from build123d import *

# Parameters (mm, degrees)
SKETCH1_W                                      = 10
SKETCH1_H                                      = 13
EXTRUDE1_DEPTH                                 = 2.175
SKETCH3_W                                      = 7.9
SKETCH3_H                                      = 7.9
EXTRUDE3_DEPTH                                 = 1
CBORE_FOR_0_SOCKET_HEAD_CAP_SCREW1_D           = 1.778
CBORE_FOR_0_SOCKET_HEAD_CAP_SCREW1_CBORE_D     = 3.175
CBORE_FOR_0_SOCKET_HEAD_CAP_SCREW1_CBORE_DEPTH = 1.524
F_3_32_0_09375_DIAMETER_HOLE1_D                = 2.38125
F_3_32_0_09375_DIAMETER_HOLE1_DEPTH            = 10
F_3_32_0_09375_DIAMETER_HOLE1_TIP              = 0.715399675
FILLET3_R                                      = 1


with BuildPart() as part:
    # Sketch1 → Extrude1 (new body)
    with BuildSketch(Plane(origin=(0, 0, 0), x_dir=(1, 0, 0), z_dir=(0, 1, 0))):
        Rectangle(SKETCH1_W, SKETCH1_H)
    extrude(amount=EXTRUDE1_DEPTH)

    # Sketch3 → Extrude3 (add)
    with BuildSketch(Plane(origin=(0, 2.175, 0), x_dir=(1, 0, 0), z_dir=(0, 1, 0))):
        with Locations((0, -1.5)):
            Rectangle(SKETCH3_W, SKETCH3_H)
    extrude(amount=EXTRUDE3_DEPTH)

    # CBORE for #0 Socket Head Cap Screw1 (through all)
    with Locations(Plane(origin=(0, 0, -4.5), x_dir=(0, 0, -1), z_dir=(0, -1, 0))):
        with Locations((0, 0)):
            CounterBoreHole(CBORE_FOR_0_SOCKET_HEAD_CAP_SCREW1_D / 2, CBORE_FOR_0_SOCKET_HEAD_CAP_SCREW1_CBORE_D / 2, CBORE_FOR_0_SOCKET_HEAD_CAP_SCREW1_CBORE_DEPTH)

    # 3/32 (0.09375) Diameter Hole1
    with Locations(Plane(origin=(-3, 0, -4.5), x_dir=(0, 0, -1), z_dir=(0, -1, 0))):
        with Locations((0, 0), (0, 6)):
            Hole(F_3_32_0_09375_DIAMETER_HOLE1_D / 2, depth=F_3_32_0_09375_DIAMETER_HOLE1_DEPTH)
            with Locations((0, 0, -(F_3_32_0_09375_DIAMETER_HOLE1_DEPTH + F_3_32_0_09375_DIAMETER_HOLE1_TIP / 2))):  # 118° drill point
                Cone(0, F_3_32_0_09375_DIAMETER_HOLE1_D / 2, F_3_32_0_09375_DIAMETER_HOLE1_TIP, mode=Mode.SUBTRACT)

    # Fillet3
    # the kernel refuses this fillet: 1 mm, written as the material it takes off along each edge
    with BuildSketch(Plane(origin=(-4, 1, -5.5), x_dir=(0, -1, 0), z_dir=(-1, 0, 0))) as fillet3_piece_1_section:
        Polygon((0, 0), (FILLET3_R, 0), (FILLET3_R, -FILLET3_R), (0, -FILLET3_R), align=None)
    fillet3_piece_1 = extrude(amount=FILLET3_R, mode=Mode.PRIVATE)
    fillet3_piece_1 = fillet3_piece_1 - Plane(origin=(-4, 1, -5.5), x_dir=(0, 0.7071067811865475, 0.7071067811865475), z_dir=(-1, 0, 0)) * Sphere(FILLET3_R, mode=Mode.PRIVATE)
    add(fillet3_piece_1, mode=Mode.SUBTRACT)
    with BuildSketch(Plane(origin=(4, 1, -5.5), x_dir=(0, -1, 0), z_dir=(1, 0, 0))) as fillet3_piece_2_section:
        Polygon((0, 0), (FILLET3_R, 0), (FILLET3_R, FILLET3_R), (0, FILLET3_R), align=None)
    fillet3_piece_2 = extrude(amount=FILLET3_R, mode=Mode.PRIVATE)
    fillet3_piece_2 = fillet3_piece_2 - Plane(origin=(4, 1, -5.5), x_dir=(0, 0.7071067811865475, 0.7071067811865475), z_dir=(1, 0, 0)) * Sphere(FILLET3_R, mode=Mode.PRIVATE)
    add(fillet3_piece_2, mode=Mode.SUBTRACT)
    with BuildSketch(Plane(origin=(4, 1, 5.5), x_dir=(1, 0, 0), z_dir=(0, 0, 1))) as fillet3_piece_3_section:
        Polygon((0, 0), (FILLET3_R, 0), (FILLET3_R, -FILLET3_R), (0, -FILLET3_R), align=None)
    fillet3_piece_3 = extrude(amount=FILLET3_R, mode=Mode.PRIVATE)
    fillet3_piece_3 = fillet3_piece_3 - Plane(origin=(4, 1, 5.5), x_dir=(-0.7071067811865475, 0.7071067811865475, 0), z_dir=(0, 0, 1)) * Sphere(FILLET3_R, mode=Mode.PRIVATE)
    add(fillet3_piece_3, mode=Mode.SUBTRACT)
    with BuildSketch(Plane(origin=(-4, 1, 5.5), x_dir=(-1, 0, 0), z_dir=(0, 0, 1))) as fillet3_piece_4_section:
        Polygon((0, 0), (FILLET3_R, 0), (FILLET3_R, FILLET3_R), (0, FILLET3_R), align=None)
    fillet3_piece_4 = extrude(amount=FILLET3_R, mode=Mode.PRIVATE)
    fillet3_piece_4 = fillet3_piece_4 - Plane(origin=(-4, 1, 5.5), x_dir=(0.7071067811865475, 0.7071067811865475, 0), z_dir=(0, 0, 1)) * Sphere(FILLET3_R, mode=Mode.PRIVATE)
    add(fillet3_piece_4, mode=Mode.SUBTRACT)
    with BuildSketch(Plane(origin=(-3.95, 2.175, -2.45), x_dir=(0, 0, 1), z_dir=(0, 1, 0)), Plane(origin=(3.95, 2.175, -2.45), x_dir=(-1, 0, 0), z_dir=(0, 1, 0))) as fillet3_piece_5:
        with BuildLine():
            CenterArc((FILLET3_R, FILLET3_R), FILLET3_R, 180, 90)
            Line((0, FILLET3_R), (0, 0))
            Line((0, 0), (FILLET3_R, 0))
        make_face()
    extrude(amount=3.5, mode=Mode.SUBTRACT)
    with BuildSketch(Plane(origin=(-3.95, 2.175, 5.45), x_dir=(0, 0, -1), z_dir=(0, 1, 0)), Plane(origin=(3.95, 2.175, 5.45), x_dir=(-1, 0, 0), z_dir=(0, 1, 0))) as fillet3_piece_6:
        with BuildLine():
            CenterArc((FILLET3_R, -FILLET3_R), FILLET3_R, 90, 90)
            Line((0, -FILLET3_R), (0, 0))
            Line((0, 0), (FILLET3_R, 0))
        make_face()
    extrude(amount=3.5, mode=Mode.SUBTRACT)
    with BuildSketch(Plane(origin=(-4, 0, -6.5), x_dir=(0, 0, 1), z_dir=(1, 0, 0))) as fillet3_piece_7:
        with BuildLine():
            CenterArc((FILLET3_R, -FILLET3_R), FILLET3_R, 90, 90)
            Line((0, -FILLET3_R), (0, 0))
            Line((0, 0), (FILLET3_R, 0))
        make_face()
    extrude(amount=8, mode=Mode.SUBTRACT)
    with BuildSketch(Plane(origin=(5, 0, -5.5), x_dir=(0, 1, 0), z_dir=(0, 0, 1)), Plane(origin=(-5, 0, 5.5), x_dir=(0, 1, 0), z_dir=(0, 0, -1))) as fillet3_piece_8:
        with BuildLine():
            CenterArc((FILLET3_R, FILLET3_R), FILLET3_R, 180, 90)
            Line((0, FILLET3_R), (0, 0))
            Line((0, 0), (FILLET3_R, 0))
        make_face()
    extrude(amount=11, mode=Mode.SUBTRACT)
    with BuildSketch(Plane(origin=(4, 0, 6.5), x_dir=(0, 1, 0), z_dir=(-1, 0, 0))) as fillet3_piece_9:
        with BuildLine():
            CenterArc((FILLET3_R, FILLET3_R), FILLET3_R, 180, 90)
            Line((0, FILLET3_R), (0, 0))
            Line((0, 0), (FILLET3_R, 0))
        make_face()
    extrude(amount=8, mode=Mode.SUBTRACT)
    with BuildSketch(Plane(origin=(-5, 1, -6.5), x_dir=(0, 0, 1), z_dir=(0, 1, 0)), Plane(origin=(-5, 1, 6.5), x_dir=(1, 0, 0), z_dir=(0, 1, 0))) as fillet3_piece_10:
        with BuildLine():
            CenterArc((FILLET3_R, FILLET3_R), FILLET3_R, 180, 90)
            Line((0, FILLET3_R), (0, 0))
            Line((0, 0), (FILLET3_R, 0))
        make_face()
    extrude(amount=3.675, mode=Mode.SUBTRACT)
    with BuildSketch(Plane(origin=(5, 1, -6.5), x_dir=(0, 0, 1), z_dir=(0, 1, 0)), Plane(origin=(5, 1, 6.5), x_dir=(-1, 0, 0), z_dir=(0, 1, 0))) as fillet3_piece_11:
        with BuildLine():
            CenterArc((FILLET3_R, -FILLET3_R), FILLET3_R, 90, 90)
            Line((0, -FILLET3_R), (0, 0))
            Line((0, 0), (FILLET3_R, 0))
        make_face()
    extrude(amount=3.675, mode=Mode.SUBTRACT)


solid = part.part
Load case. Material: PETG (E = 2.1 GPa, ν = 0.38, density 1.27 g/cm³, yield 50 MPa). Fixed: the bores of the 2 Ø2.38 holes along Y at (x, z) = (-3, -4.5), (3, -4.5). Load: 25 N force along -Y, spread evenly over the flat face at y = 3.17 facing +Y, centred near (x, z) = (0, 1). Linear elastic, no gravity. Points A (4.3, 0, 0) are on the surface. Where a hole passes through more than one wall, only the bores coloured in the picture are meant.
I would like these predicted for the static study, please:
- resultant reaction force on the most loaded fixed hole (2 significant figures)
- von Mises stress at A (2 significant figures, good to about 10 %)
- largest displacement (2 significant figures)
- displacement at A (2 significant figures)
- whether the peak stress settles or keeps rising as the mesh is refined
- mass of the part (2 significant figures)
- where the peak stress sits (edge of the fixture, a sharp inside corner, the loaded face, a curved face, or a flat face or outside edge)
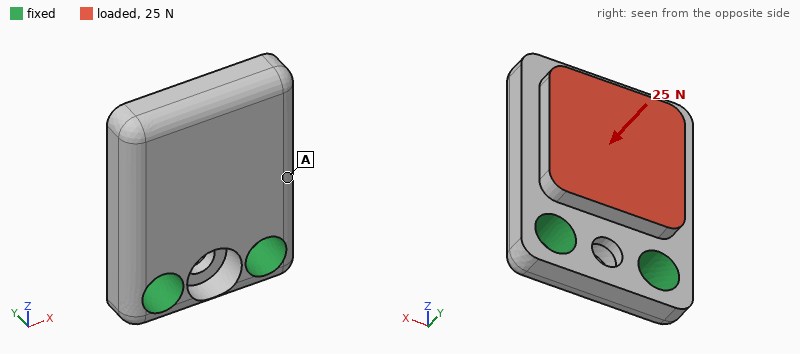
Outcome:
13 N
4.0 MPa
0.17 mm
0.049 mm
keeps rising
0.38 g
edge of the fixture
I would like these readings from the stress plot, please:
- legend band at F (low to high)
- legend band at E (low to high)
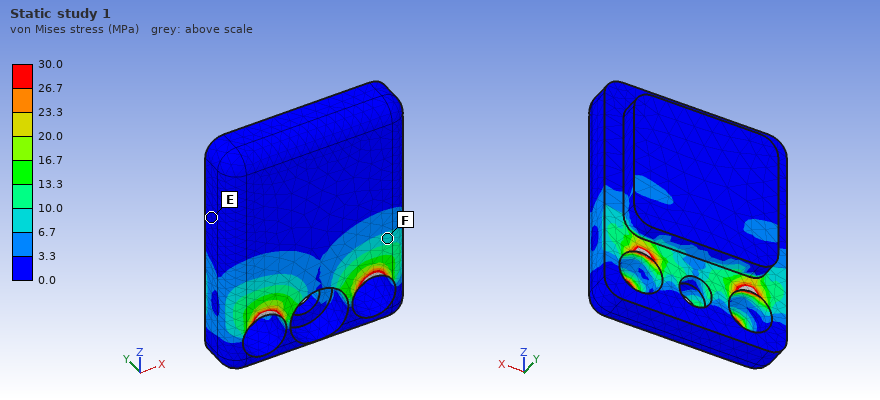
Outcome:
6.7 to 10.0 MPa
0.0 to 3.3 MPa
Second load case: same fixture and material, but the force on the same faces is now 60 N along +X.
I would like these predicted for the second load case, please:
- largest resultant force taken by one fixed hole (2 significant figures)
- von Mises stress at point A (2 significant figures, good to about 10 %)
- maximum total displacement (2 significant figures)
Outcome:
56 N
1.8 MPa
58 µm
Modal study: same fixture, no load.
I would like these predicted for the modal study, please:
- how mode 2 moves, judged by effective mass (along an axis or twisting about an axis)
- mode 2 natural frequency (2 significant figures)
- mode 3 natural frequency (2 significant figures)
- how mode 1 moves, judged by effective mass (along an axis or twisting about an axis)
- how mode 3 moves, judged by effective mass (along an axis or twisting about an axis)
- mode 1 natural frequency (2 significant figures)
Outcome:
along X
11 kHz
12 kHz
along Y
along X
4100 Hz
